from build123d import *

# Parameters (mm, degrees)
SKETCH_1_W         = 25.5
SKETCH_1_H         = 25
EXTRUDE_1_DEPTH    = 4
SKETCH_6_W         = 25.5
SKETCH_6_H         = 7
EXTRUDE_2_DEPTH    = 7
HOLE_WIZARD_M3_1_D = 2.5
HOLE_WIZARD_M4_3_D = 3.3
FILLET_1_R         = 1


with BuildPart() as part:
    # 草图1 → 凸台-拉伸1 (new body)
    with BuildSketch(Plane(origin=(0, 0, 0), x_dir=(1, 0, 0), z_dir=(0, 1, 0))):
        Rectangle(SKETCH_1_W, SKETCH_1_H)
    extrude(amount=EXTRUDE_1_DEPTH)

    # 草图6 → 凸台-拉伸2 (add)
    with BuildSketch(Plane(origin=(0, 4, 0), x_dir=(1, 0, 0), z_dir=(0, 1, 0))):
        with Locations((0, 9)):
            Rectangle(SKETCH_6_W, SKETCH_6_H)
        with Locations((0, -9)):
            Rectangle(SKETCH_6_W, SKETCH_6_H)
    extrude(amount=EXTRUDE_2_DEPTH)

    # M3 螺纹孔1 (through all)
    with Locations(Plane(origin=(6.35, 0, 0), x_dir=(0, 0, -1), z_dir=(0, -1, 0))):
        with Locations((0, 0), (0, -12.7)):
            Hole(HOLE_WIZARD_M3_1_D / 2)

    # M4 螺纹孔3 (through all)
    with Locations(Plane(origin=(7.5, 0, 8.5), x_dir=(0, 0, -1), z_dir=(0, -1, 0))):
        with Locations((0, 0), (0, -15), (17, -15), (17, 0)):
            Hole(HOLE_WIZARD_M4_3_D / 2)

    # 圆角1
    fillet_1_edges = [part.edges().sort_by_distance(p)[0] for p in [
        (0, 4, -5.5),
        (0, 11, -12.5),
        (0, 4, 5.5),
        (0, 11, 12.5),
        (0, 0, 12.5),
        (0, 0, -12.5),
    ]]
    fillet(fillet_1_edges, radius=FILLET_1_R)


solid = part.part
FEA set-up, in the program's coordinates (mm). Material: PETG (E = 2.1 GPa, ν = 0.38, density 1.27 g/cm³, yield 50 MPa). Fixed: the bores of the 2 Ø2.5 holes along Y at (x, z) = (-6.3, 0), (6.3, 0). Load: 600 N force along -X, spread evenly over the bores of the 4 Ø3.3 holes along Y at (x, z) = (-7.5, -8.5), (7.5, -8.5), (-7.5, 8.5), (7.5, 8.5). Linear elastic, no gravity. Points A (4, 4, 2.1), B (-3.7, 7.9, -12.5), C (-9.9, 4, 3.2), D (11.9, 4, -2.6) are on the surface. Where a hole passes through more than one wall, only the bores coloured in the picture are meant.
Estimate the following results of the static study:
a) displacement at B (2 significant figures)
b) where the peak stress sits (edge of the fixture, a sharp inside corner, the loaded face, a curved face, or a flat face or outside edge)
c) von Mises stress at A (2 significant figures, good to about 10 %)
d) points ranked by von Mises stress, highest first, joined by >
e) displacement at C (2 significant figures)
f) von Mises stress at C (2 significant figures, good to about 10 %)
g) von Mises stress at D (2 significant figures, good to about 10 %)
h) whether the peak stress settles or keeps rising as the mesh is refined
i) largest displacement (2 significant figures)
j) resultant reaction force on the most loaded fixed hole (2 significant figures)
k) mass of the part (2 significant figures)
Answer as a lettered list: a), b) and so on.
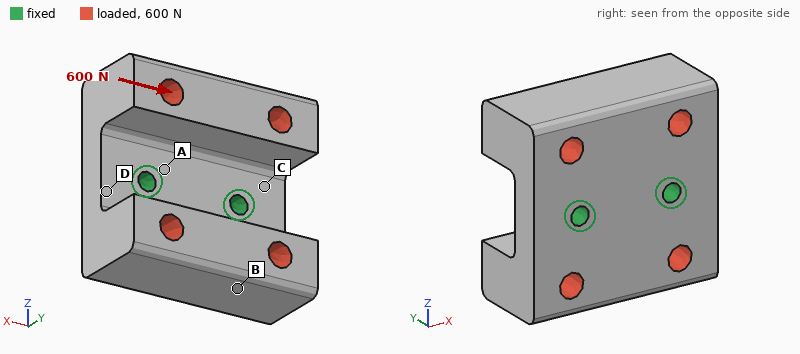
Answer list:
a) 0.075 mm
b) edge of the fixture
c) 9.9 MPa
d) A > C > D > B
e) 0.036 mm
f) 6.6 MPa
g) 3.8 MPa
h) keeps rising
i) 0.12 mm
j) 330 N
k) 5.9 g
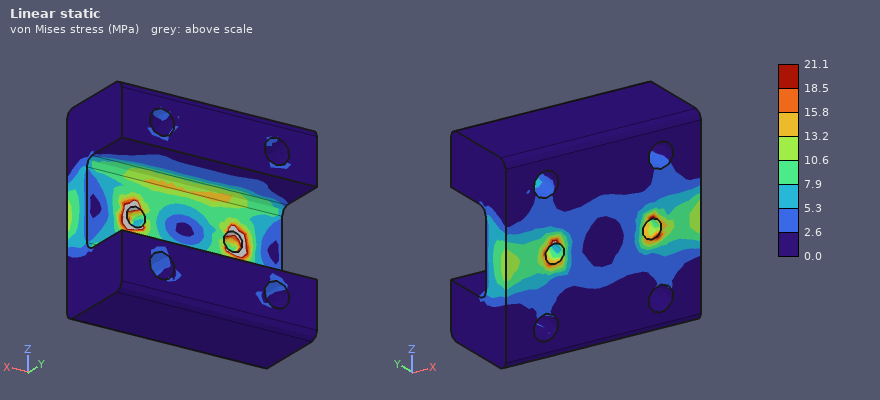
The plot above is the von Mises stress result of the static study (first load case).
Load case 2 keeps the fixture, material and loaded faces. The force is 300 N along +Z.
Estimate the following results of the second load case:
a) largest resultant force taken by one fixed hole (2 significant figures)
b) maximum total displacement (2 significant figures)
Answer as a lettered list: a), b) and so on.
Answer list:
a) 150 N
b) 0.20 mm
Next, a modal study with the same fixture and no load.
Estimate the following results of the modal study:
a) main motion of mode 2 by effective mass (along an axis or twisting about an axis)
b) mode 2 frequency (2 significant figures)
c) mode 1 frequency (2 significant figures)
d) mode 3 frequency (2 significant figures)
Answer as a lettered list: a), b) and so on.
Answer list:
a) along Y
b) 2900 Hz
c) 2300 Hz
d) 4600 Hz
